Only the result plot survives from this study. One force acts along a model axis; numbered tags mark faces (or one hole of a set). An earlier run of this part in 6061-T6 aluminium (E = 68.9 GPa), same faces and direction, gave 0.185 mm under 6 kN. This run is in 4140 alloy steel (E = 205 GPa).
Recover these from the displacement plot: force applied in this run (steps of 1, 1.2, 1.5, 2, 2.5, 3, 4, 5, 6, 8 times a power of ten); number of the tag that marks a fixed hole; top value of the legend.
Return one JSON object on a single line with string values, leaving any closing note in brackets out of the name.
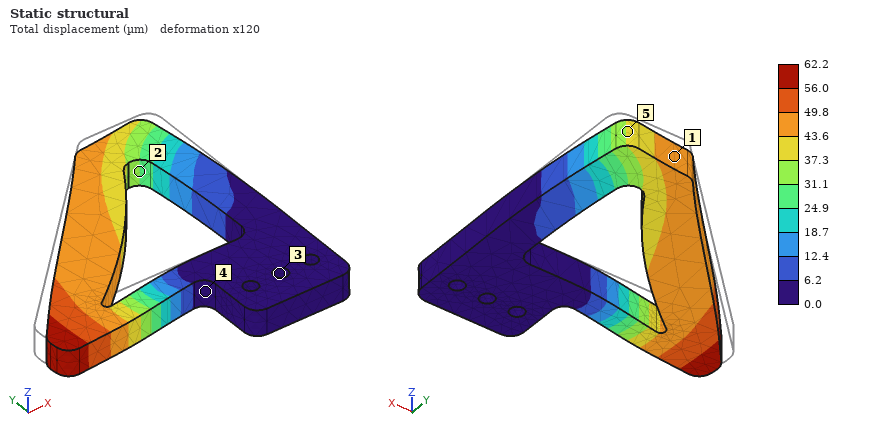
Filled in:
{"force applied in this run": "6 kN", "number of the tag that marks a fixed hole": "3", "top value of the legend": "62.2 µm"}
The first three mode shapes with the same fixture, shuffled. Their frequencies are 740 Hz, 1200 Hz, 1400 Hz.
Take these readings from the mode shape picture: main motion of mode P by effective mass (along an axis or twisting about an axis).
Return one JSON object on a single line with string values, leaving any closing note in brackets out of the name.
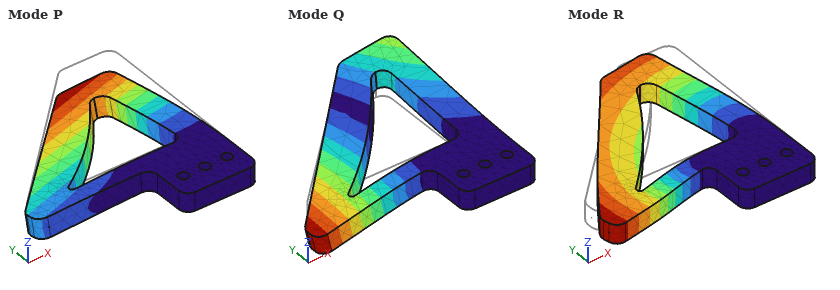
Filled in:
{"main motion of mode P by effective mass": "along Z"}
